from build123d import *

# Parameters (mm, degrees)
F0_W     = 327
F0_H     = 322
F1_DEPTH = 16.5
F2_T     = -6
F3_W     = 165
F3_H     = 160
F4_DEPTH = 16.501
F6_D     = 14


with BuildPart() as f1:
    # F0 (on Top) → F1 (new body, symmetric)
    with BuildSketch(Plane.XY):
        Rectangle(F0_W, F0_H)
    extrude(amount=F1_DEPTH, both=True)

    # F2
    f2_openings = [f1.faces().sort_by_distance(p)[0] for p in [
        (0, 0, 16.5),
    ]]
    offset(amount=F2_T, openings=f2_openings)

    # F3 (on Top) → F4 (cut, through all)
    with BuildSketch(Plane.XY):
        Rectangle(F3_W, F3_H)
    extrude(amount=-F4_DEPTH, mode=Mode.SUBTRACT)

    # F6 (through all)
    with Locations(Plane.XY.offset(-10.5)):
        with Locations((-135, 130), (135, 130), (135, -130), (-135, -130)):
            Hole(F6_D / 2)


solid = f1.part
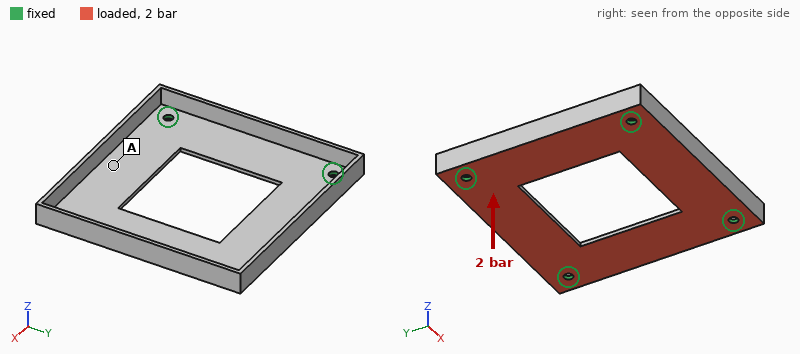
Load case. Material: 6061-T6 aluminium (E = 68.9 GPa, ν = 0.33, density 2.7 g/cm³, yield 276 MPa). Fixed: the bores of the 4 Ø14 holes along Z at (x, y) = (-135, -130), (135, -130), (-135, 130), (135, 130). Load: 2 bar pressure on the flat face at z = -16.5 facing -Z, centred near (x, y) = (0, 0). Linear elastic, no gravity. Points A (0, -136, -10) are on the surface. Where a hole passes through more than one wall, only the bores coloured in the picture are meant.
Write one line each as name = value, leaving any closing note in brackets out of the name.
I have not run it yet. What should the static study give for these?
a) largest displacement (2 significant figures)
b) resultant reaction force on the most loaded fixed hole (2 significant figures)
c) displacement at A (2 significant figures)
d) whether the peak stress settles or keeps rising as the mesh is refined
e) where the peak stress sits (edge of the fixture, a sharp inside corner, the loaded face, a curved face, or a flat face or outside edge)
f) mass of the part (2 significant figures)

largest displacement = 1.9 mm
resultant reaction force on the most loaded fixed hole = 4.5 kN
displacement at A = 0.62 mm
whether the peak stress settles or keeps rising as the mesh is refined = keeps rising
where the peak stress sits = edge of the fixture
mass of the part = 1.8 kg
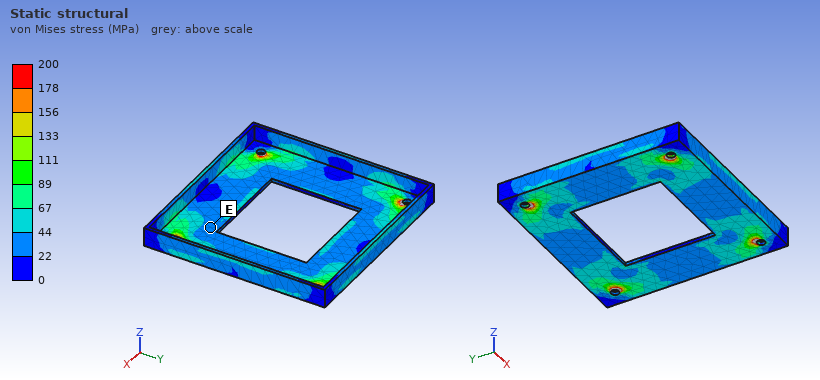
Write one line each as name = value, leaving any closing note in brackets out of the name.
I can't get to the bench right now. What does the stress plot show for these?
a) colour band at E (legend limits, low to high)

colour band at E = 22 to 44 MPa
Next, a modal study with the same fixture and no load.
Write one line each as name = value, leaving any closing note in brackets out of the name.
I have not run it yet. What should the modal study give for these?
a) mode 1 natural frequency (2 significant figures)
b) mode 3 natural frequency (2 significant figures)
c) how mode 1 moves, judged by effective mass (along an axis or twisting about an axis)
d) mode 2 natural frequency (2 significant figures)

mode 1 natural frequency = 540 Hz
mode 3 natural frequency = 720 Hz
how mode 1 moves, judged by effective mass = along Z
mode 2 natural frequency = 700 Hz
